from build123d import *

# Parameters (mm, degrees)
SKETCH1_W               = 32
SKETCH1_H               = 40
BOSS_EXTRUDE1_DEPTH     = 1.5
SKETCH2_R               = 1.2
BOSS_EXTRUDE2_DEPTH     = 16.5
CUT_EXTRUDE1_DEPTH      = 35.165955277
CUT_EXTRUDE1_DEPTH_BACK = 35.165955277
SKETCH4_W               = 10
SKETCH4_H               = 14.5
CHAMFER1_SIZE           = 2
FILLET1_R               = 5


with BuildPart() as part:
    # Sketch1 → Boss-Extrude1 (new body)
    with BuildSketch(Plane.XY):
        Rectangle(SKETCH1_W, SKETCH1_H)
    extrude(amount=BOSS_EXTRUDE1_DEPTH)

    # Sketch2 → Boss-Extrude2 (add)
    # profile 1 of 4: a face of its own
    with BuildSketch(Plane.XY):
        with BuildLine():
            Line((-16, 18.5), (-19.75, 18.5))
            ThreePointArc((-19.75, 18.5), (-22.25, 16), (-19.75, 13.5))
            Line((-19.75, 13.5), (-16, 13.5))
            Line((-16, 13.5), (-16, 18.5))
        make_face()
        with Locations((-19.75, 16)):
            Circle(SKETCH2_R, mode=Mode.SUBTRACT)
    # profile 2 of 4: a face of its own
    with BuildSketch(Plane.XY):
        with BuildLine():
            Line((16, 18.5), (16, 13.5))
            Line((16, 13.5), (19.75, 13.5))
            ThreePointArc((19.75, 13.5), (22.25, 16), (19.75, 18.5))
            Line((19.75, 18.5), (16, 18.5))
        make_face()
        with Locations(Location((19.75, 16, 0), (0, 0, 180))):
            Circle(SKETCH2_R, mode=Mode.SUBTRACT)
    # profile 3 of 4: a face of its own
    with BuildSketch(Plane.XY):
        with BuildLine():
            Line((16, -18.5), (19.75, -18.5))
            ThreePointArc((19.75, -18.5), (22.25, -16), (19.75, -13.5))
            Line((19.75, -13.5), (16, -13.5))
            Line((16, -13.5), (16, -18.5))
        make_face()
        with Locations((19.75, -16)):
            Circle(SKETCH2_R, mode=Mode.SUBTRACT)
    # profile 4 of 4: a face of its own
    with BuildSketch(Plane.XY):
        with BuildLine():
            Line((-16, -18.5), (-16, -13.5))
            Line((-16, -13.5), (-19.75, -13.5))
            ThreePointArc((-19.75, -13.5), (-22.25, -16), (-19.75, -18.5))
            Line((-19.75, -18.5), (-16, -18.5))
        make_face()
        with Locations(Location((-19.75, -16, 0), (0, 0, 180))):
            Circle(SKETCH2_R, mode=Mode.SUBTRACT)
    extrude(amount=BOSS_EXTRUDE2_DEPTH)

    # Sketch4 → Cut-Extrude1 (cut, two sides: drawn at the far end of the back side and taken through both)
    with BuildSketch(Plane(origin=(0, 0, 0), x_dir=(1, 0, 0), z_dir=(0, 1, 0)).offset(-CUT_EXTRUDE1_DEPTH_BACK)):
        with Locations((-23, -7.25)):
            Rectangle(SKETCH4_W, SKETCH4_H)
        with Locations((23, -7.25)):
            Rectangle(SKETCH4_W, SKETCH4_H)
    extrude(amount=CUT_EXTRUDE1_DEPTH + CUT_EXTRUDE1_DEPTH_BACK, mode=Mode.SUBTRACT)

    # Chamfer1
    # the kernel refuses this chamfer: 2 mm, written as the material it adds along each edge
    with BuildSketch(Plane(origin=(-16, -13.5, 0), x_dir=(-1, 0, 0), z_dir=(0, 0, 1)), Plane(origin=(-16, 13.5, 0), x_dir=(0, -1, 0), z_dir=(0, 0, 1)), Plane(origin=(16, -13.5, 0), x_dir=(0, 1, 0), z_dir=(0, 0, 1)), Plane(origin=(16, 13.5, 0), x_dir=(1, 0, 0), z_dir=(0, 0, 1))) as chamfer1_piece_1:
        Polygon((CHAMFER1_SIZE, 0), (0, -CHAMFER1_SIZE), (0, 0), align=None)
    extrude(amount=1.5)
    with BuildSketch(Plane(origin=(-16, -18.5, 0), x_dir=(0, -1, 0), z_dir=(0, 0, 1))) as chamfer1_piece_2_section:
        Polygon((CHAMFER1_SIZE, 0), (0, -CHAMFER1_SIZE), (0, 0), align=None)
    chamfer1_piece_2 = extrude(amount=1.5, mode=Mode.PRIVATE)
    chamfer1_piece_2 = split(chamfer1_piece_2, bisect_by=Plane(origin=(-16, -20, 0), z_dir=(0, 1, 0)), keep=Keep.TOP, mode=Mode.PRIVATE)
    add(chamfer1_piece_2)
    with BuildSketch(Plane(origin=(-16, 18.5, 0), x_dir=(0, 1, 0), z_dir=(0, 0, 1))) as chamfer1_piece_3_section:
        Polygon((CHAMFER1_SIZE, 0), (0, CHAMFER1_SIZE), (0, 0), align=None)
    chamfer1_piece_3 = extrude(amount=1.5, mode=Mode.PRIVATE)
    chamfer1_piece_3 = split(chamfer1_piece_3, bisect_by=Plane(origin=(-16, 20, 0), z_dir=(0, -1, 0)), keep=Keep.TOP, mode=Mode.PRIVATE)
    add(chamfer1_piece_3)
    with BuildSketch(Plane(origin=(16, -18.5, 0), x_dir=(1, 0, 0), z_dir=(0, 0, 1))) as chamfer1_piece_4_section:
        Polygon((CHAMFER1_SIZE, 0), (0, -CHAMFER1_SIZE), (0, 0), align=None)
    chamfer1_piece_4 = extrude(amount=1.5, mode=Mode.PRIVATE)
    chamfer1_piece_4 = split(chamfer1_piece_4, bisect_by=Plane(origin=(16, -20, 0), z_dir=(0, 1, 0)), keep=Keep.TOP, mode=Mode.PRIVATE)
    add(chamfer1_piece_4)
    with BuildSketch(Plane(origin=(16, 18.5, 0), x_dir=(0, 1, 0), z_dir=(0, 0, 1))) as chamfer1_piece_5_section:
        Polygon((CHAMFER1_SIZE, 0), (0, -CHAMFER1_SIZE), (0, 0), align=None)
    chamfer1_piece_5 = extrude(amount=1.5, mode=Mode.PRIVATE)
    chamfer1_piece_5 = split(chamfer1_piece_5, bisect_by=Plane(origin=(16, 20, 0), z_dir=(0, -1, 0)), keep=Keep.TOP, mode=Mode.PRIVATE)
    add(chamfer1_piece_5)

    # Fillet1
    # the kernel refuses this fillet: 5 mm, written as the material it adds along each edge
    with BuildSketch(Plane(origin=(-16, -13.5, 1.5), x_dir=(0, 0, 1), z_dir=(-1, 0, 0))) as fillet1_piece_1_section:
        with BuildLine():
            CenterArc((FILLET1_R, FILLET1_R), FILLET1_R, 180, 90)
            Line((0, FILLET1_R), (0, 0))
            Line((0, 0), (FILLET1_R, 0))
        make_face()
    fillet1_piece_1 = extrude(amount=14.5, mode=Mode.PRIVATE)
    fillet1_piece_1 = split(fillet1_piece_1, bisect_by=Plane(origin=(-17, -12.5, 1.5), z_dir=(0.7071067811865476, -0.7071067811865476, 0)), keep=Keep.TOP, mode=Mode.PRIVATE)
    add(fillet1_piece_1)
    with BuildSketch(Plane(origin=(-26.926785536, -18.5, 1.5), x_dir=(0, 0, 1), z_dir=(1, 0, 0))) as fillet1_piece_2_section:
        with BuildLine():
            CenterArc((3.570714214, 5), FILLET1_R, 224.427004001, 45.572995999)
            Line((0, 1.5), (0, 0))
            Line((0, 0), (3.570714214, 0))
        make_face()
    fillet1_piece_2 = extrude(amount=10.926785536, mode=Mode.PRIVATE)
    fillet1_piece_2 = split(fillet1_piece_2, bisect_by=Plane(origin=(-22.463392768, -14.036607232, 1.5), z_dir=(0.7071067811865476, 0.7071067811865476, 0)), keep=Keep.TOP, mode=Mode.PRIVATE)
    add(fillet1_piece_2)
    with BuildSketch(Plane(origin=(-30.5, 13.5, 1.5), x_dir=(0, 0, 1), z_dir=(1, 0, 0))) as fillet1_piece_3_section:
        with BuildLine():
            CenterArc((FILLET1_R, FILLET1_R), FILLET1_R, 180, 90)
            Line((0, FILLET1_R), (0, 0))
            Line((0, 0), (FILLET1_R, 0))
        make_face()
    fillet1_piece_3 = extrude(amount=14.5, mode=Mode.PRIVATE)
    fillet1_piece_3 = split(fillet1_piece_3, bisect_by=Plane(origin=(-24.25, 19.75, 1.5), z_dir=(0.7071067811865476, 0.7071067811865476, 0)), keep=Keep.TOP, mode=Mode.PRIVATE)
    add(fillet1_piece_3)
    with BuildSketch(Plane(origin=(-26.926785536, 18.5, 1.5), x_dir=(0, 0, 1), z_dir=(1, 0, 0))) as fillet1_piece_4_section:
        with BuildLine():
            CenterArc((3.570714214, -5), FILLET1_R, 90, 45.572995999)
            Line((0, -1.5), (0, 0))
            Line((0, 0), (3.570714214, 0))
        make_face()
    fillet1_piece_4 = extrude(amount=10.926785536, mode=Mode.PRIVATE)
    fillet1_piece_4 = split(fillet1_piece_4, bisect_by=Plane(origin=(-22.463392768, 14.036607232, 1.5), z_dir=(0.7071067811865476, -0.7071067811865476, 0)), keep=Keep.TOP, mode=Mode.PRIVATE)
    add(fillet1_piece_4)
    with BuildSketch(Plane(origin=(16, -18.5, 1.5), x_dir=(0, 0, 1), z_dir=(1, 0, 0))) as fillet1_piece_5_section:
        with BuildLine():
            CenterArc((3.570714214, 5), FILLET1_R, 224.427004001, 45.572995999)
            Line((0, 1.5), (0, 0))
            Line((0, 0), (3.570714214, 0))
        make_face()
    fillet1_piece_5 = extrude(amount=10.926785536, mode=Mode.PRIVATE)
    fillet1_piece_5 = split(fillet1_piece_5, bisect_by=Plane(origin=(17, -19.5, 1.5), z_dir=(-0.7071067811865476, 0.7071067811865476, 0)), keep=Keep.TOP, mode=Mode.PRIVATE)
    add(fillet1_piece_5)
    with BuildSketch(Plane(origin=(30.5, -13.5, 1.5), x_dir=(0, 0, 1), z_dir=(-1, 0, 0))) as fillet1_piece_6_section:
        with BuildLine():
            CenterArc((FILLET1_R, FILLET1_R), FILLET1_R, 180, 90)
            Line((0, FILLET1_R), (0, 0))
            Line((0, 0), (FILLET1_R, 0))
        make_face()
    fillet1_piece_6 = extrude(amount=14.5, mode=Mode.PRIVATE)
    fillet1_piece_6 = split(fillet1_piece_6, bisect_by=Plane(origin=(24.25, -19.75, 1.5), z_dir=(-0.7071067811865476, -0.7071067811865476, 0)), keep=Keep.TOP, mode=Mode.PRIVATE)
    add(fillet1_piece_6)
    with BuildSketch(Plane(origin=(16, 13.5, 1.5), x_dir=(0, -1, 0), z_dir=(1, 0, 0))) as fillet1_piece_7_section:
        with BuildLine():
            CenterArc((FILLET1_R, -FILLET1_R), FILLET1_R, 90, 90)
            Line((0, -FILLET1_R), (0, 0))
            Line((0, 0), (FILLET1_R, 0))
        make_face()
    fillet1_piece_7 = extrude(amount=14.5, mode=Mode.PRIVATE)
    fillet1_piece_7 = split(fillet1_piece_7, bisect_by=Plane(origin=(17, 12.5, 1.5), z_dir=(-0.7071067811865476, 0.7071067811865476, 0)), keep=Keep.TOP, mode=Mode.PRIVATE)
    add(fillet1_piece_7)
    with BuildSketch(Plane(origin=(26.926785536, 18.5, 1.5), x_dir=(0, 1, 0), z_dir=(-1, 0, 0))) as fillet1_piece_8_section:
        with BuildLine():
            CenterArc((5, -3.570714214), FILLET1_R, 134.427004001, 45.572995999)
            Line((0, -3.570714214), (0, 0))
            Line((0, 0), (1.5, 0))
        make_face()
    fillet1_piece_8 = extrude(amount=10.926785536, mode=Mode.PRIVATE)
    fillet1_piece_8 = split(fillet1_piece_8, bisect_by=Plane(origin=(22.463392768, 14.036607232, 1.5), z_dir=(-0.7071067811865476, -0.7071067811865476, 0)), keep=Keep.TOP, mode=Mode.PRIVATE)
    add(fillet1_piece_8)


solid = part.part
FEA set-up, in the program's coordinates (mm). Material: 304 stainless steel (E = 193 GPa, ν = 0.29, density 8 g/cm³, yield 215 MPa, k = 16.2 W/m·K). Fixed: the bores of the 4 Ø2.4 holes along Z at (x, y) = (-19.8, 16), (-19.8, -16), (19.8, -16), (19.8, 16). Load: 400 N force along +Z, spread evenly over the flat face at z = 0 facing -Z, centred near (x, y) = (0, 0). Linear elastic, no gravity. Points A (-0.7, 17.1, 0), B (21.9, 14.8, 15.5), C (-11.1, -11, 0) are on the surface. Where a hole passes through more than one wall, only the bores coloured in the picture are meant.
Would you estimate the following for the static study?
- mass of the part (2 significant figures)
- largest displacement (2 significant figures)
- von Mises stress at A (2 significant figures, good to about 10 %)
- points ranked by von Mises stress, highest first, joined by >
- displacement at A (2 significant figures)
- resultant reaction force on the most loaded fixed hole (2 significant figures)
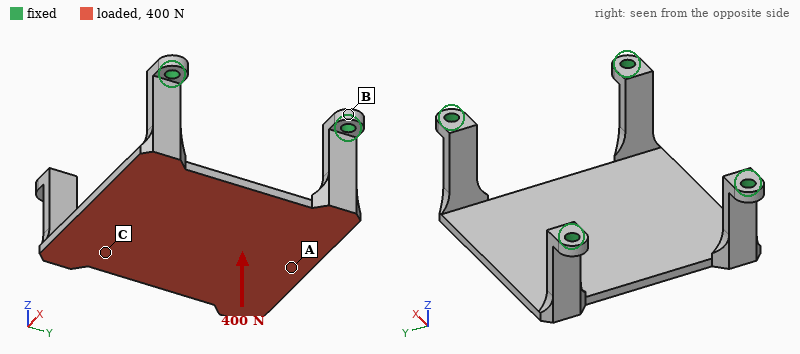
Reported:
22 g
53 µm
63 MPa
A > C > B
40 µm
110 N
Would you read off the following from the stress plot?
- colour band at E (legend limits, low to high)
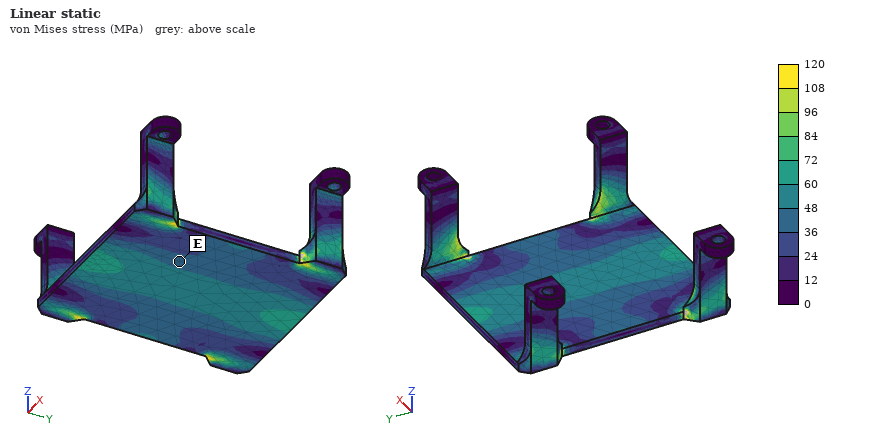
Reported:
36 to 48 MPa
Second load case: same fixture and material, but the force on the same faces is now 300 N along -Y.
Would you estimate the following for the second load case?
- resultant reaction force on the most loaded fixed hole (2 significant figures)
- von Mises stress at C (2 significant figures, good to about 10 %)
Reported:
78 N
38 MPa
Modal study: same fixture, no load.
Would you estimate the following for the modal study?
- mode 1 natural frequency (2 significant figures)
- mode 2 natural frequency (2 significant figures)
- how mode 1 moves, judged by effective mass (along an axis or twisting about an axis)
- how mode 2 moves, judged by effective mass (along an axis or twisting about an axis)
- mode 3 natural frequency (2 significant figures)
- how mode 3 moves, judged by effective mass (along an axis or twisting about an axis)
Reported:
2500 Hz
3700 Hz
along X
along Y
4100 Hz
along Z
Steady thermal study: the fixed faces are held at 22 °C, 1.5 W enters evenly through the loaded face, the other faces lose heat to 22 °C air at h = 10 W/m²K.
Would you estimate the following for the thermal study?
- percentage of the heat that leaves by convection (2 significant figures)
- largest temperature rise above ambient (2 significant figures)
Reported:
37 %
32 K
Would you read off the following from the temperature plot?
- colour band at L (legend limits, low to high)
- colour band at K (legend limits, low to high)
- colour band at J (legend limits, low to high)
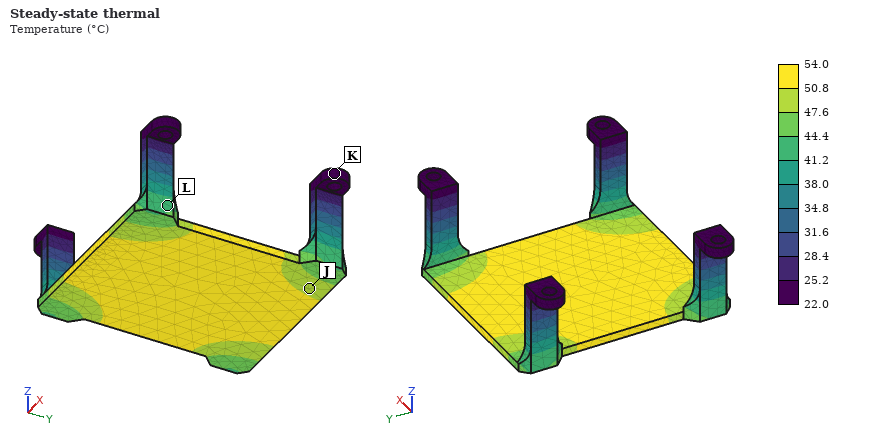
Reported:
41.2 to 44.4 °C
22.0 to 25.2 °C
47.6 to 50.8 °C
